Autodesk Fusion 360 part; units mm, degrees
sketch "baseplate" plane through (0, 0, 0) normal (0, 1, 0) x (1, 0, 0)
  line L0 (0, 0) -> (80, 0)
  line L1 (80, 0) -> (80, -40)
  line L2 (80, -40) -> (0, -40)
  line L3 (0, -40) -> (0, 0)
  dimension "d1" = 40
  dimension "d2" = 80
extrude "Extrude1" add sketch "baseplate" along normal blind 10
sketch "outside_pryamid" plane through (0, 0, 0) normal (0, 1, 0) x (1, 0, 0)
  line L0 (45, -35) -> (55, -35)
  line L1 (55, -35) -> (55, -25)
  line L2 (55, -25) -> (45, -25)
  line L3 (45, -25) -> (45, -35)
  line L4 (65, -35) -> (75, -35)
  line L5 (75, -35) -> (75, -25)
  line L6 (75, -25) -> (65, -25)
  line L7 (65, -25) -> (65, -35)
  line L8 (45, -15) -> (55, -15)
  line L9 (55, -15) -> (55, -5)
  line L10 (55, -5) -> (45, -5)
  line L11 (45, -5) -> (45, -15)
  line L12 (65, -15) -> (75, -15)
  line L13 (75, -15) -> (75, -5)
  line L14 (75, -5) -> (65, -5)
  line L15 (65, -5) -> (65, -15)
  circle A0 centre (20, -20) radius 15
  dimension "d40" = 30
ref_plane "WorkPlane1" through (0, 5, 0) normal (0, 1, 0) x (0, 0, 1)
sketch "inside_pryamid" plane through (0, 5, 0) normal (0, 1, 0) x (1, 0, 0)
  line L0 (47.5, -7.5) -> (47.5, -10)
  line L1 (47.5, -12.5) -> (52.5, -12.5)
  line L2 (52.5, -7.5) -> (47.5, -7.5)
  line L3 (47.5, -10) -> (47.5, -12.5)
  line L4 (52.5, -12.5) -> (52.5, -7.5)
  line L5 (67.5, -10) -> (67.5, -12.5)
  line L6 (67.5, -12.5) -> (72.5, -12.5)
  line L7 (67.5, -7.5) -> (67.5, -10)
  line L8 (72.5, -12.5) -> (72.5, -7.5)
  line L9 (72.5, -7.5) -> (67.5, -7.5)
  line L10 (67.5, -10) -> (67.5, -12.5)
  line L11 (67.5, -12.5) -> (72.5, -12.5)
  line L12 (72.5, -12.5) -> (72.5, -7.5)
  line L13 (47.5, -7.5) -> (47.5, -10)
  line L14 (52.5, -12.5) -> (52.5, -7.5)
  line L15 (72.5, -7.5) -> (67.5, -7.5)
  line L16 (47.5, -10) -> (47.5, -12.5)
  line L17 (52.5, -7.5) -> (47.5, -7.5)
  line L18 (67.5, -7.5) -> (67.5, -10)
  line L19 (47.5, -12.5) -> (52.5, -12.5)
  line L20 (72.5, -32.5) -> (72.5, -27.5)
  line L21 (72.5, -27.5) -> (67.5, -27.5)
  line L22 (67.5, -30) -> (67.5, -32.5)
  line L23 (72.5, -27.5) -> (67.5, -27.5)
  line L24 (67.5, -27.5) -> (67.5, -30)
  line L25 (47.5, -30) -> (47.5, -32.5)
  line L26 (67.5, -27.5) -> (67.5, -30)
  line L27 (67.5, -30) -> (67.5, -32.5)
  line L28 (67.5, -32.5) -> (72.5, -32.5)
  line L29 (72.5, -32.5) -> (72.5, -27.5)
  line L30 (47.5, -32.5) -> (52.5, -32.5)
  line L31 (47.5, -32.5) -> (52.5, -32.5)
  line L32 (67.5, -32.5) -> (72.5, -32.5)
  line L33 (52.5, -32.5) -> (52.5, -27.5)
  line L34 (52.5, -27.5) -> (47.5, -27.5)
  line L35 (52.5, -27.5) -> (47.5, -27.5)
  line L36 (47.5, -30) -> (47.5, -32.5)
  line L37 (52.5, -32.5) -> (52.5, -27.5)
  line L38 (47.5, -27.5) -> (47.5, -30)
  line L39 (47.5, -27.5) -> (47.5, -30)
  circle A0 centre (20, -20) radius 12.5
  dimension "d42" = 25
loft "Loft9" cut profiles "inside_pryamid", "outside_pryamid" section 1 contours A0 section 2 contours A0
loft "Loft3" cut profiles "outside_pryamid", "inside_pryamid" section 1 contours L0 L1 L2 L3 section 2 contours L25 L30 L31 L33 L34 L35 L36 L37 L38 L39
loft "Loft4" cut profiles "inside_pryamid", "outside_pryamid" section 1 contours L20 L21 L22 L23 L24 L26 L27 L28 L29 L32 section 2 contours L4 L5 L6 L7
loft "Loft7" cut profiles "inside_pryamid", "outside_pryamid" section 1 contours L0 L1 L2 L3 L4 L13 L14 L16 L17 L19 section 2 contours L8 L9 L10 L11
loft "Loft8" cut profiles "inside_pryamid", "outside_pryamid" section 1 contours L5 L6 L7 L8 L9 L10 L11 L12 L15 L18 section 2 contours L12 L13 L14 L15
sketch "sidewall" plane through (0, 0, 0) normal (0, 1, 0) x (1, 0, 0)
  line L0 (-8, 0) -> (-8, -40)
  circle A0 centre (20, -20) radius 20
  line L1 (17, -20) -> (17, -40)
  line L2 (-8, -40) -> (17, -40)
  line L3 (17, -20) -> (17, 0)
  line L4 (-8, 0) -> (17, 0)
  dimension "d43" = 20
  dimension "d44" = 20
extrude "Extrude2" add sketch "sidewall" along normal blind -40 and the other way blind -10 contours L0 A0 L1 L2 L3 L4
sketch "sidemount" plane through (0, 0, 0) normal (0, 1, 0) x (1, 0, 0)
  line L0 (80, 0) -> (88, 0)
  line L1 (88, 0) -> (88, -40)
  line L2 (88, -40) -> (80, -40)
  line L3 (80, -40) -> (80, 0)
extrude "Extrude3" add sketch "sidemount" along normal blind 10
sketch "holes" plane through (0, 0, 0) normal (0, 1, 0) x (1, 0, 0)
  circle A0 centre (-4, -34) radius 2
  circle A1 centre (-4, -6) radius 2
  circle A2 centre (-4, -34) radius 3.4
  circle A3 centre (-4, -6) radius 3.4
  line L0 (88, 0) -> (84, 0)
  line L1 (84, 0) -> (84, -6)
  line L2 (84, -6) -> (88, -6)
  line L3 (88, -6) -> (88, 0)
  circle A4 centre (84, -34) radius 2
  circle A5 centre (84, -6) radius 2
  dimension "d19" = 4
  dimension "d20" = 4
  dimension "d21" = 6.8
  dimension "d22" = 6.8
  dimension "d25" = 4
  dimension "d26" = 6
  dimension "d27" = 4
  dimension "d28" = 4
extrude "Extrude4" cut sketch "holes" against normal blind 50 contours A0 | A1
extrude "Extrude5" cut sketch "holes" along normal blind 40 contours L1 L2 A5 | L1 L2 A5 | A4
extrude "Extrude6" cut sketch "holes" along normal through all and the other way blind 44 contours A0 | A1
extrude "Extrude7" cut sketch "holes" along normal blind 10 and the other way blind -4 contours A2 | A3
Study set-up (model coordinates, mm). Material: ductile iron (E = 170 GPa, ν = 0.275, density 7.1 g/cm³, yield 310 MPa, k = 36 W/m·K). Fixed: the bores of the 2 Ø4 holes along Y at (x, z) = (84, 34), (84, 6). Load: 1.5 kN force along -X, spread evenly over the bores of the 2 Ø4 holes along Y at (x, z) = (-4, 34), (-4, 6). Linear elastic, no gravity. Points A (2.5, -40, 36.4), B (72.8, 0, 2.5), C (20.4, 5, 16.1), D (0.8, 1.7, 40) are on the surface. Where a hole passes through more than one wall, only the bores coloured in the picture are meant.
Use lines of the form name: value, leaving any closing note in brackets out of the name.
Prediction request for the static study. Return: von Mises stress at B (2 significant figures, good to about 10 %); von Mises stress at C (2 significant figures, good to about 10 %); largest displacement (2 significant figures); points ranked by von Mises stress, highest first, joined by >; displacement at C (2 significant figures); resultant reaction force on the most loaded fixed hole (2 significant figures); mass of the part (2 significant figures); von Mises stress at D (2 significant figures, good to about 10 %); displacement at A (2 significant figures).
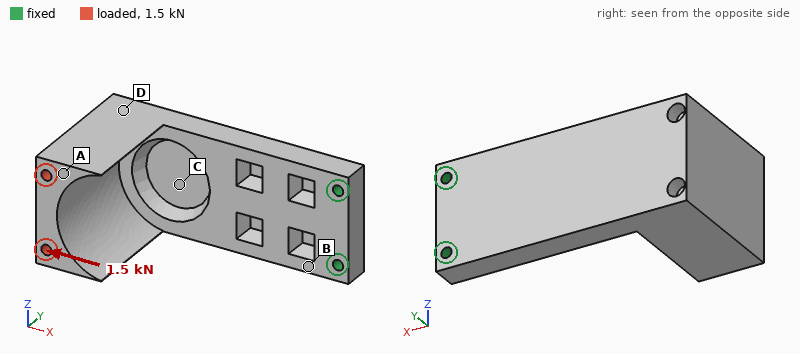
von Mises stress at B: 85 MPa
von Mises stress at C: 44 MPa
largest displacement: 0.50 mm
points ranked by von Mises stress, highest first, joined by >: B > C > D > A
displacement at C: 0.17 mm
resultant reaction force on the most loaded fixed hole: 750 N
mass of the part: 370 g
von Mises stress at D: 31 MPa
displacement at A: 0.45 mm
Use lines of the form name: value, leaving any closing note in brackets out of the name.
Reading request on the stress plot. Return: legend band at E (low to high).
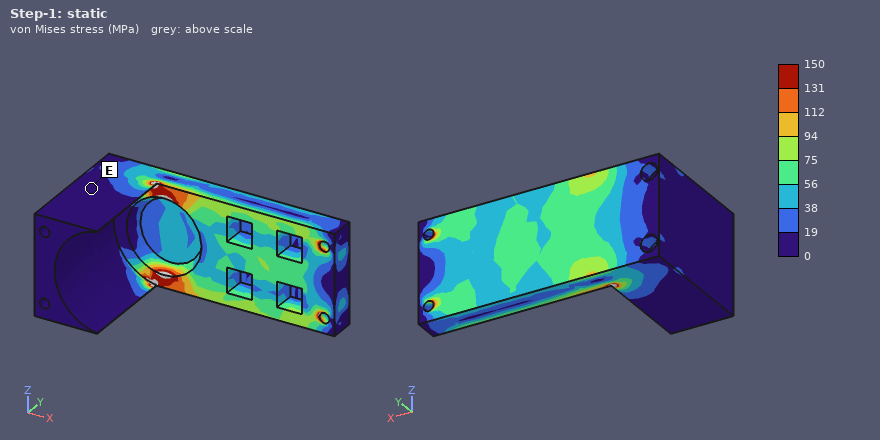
legend band at E: 0 to 19 MPa
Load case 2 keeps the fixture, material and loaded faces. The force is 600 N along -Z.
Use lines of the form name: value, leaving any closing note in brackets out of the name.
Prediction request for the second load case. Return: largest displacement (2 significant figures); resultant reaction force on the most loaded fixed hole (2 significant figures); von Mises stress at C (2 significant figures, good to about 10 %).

largest displacement: 0.11 mm
resultant reaction force on the most loaded fixed hole: 1.9 kN
von Mises stress at C: 22 MPa
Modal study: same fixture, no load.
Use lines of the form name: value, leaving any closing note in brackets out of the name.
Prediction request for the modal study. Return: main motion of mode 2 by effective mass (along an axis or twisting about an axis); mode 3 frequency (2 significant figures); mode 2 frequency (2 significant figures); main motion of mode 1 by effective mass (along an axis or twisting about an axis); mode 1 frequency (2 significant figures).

main motion of mode 2 by effective mass: along Z
mode 3 frequency: 1900 Hz
mode 2 frequency: 1100 Hz
main motion of mode 1 by effective mass: along Y
mode 1 frequency: 470 Hz
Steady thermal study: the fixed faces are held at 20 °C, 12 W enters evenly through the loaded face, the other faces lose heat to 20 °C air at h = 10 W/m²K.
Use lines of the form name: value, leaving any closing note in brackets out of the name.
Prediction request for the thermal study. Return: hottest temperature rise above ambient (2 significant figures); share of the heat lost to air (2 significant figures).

hottest temperature rise above ambient: 58 K
share of the heat lost to air: 49 %
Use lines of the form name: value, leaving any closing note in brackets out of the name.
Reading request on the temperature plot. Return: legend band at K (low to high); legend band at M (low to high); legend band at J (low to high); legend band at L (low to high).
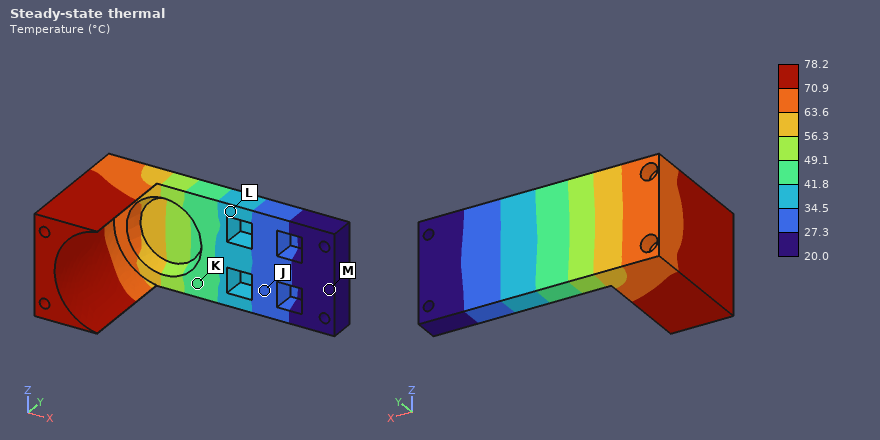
legend band at K: 41.8 to 49.1 °C
legend band at M: 20.0 to 27.3 °C
legend band at J: 27.3 to 34.5 °C
legend band at L: 34.5 to 41.8 °C
